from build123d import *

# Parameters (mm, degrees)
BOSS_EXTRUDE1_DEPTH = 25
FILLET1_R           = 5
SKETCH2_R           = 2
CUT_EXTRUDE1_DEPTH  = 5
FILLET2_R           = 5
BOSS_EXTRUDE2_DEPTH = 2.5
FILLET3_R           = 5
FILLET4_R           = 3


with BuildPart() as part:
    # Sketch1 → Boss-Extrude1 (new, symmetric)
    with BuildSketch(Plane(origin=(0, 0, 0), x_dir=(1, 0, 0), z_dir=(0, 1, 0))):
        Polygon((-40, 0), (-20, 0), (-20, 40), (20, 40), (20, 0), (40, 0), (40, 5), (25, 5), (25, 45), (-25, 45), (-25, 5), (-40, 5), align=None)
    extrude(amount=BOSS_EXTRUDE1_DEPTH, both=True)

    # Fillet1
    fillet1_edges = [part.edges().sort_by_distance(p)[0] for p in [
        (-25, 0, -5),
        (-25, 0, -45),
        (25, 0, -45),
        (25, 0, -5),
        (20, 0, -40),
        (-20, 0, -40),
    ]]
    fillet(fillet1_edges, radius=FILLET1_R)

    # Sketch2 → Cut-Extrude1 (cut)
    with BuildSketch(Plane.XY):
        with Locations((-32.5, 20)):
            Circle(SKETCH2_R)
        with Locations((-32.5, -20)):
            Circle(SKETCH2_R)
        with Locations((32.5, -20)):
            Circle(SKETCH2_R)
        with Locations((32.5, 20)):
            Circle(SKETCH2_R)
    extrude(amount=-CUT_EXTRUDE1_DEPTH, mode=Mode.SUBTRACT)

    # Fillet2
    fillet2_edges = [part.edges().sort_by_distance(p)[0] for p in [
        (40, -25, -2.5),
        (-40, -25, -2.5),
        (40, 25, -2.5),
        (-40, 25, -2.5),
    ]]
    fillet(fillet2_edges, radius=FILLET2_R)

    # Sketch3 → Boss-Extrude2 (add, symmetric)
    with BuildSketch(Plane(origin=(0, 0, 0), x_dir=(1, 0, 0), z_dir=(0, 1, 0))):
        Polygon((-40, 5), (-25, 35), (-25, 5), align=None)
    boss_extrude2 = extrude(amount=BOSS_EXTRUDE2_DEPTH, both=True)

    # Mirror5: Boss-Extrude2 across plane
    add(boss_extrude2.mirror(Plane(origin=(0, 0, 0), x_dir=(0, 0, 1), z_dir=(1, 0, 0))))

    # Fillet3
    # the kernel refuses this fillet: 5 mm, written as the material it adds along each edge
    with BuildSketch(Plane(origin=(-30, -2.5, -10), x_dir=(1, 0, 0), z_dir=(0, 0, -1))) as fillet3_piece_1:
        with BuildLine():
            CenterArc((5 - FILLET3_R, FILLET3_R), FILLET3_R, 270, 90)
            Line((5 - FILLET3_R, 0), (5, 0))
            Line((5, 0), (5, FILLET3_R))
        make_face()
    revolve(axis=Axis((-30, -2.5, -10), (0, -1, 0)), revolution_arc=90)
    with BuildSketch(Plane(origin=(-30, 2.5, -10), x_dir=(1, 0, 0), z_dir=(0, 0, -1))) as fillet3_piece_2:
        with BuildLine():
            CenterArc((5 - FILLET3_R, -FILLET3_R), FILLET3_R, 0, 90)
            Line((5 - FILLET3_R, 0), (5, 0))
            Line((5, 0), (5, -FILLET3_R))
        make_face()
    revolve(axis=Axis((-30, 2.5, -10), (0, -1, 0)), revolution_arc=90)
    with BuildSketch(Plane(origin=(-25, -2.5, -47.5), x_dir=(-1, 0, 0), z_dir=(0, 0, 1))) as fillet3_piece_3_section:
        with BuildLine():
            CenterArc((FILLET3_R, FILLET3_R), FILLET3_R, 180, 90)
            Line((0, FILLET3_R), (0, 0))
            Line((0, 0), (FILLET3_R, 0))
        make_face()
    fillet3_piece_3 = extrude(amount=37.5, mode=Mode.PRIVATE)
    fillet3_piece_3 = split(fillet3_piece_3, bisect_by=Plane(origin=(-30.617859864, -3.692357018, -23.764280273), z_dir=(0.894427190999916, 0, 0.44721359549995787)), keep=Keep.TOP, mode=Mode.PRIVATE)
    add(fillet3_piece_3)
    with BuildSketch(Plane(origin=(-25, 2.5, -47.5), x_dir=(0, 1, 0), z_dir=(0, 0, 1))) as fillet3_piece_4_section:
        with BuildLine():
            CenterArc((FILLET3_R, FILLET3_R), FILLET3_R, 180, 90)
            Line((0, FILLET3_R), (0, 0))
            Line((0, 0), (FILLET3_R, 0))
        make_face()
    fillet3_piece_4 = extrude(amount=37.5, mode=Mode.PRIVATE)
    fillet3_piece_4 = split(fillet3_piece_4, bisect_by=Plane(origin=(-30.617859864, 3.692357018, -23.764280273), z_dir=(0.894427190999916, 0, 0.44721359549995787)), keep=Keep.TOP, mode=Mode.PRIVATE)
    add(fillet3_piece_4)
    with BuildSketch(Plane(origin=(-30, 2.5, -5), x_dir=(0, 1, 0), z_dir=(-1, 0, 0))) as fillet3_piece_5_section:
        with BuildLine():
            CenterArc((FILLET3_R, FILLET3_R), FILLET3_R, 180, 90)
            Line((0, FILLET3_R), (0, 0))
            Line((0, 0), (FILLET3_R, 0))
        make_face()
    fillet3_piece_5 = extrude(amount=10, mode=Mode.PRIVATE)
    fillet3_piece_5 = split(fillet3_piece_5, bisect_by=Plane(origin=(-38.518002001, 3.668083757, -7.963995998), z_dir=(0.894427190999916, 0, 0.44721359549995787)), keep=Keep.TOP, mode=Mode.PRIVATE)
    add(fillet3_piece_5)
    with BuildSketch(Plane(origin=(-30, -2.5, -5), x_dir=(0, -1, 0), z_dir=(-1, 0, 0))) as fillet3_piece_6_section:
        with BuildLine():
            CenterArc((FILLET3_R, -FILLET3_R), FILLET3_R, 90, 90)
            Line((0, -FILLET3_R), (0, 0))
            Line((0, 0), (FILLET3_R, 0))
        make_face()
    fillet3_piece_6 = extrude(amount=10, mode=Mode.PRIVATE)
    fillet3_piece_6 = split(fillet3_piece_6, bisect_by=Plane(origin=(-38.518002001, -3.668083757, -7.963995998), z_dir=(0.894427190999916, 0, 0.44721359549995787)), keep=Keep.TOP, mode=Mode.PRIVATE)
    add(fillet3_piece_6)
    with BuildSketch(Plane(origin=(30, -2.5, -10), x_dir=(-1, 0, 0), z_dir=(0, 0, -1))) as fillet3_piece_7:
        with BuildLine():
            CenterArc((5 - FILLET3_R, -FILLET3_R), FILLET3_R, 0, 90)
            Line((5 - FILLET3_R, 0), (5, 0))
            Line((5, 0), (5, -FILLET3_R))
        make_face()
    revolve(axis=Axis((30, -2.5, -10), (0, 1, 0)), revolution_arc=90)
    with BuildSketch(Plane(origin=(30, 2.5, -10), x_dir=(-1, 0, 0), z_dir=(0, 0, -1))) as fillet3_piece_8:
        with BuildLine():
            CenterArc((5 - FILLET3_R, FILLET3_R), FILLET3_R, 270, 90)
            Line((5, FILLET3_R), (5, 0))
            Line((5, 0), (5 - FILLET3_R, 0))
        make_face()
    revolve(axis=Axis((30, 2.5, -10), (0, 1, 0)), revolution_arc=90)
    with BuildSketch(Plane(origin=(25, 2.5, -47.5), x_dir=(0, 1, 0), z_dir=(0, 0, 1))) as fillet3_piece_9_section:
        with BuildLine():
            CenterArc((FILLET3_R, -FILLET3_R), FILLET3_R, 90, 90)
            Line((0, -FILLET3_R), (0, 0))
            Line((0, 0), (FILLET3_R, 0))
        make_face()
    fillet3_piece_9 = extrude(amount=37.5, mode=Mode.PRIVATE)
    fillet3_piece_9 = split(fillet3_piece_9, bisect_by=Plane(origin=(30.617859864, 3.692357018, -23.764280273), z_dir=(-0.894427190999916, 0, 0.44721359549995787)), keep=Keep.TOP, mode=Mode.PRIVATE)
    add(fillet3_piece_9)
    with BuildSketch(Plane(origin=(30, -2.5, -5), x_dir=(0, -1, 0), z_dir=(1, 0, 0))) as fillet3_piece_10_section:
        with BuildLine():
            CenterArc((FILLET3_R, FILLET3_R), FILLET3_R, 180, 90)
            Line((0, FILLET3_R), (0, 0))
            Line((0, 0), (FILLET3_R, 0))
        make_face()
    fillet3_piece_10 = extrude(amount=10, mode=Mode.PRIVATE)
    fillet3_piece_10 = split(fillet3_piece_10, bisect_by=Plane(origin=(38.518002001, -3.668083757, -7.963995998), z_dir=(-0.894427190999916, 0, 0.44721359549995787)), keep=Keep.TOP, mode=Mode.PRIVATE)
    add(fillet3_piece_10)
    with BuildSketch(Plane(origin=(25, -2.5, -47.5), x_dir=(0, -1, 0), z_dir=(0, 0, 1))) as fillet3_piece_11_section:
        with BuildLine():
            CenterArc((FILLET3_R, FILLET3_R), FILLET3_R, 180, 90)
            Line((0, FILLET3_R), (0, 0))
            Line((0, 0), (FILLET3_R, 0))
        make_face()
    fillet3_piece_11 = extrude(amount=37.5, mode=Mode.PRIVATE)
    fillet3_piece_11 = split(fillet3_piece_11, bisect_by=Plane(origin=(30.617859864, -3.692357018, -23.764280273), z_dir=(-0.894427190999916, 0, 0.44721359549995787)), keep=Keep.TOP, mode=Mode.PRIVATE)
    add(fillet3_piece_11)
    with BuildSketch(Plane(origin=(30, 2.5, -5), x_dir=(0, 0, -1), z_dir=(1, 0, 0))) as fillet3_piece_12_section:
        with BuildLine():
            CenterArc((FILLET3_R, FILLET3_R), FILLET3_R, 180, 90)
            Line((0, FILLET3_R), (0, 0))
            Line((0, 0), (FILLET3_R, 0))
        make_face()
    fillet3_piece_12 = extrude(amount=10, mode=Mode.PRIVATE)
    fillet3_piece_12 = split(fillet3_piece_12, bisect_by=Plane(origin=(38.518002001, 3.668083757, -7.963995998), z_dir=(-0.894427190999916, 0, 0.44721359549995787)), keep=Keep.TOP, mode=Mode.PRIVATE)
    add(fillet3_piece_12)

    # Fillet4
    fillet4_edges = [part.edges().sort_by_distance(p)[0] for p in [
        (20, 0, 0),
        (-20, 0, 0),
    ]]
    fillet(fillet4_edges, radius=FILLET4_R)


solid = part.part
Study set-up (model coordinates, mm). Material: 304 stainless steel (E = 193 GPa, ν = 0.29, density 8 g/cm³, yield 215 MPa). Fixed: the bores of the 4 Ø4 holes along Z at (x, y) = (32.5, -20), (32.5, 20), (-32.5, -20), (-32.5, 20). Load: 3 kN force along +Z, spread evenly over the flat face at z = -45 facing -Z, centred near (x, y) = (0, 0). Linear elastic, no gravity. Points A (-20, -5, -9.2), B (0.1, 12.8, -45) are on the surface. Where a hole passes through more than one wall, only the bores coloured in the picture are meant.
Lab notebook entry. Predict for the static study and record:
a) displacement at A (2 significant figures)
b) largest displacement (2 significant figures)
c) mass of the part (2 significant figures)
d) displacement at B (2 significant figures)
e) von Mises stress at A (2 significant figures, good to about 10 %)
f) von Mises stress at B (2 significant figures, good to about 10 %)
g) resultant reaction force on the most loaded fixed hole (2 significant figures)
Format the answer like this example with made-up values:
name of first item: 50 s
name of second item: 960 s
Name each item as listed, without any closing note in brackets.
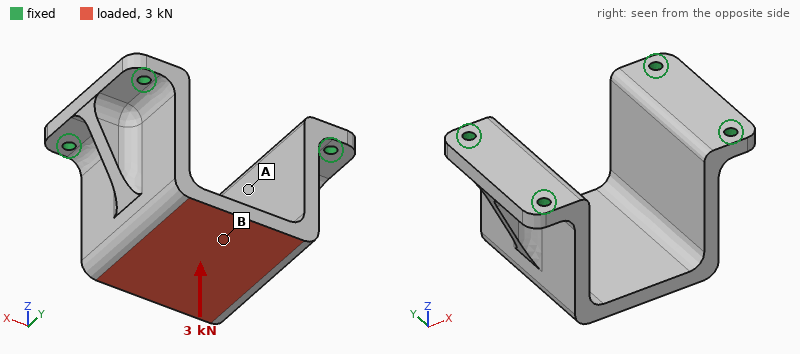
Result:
displacement at A: 2.4 µm
largest displacement: 16 µm
mass of the part: 340 g
displacement at B: 15 µm
von Mises stress at A: 7.7 MPa
von Mises stress at B: 34 MPa
resultant reaction force on the most loaded fixed hole: 820 N
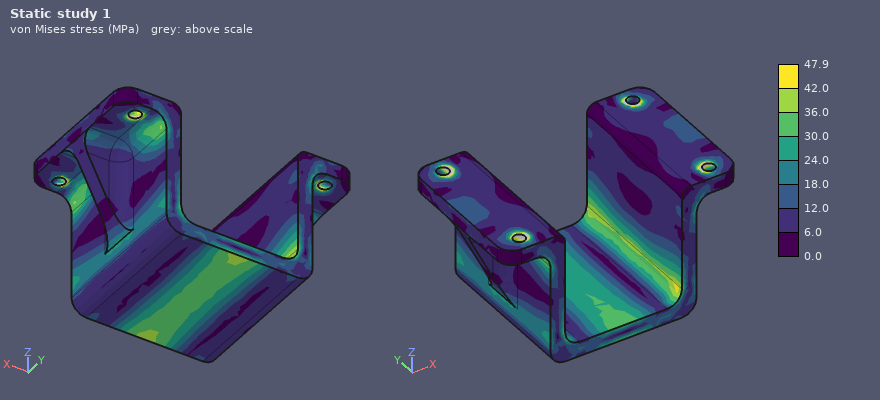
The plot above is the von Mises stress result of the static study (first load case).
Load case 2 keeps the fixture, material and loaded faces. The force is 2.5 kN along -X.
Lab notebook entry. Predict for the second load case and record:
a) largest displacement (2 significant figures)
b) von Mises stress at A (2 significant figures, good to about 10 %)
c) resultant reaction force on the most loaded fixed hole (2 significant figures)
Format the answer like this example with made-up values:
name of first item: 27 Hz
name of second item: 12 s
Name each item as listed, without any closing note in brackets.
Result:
largest displacement: 69 µm
von Mises stress at A: 22 MPa
resultant reaction force on the most loaded fixed hole: 940 N
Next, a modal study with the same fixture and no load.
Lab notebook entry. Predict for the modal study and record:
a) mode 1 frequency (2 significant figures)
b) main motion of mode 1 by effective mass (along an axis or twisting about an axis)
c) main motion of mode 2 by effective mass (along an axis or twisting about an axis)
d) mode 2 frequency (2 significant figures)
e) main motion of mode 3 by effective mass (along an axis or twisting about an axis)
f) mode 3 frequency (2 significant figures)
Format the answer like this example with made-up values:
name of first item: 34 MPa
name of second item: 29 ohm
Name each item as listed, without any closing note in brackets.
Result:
mode 1 frequency: 2400 Hz
main motion of mode 1 by effective mass: along X
main motion of mode 2 by effective mass: along Y
mode 2 frequency: 4700 Hz
main motion of mode 3 by effective mass: twisting about Z
mode 3 frequency: 5000 Hz
